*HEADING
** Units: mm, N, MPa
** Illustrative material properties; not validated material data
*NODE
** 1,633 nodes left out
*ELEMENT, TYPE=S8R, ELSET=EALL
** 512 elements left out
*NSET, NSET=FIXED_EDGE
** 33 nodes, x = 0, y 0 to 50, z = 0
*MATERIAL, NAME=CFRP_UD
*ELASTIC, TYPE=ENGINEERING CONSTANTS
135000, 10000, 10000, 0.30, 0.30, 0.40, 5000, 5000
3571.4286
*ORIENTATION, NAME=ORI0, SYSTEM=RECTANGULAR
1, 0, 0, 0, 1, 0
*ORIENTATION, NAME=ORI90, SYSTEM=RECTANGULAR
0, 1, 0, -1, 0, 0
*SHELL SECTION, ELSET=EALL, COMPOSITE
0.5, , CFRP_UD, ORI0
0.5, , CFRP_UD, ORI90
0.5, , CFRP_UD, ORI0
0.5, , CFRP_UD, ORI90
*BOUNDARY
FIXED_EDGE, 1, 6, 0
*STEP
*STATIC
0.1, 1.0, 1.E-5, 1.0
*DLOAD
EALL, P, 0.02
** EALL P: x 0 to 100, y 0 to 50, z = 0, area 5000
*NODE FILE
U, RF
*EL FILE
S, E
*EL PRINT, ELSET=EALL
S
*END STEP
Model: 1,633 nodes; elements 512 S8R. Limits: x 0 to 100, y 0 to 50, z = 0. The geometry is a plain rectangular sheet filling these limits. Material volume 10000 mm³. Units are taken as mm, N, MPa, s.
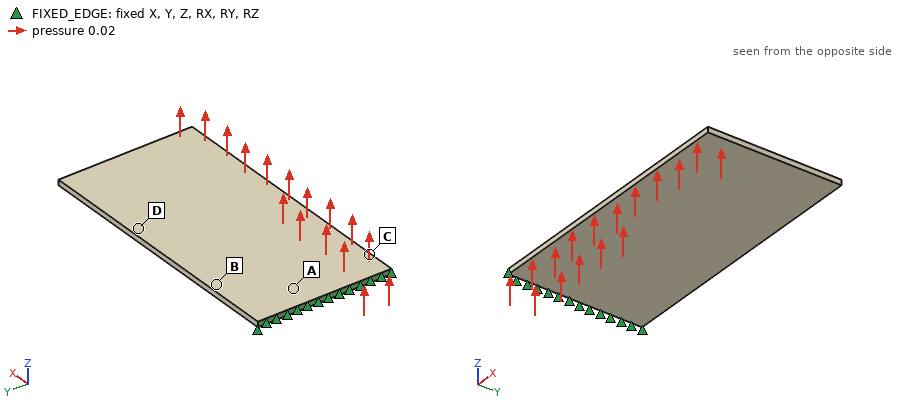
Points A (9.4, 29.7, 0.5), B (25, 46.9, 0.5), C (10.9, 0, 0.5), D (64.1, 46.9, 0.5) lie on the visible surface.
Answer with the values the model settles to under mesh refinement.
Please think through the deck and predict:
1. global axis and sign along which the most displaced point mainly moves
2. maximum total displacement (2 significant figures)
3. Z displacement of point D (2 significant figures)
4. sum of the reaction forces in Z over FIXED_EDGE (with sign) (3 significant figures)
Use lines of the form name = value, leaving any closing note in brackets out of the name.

global axis and sign along which the most displaced point mainly moves = +Z
maximum total displacement = 6.0 mm
Z displacement of point D = 3.2 mm
sum of the reaction forces in Z over FIXED_EDGE (with sign) = -100 N
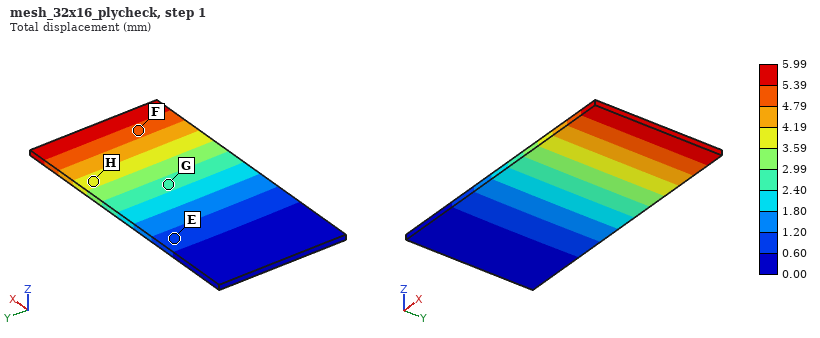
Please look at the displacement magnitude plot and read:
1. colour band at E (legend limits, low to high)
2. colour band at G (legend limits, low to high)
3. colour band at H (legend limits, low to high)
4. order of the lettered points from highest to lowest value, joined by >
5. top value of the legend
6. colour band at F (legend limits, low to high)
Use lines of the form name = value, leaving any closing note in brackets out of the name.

colour band at E = 0.60 to 1.20 mm
colour band at G = 2.40 to 2.99 mm
colour band at H = 3.59 to 4.19 mm
order of the lettered points from highest to lowest value, joined by > = F > H > G > E
top value of the legend = 5.99 mm
colour band at F = 4.79 to 5.39 mm
